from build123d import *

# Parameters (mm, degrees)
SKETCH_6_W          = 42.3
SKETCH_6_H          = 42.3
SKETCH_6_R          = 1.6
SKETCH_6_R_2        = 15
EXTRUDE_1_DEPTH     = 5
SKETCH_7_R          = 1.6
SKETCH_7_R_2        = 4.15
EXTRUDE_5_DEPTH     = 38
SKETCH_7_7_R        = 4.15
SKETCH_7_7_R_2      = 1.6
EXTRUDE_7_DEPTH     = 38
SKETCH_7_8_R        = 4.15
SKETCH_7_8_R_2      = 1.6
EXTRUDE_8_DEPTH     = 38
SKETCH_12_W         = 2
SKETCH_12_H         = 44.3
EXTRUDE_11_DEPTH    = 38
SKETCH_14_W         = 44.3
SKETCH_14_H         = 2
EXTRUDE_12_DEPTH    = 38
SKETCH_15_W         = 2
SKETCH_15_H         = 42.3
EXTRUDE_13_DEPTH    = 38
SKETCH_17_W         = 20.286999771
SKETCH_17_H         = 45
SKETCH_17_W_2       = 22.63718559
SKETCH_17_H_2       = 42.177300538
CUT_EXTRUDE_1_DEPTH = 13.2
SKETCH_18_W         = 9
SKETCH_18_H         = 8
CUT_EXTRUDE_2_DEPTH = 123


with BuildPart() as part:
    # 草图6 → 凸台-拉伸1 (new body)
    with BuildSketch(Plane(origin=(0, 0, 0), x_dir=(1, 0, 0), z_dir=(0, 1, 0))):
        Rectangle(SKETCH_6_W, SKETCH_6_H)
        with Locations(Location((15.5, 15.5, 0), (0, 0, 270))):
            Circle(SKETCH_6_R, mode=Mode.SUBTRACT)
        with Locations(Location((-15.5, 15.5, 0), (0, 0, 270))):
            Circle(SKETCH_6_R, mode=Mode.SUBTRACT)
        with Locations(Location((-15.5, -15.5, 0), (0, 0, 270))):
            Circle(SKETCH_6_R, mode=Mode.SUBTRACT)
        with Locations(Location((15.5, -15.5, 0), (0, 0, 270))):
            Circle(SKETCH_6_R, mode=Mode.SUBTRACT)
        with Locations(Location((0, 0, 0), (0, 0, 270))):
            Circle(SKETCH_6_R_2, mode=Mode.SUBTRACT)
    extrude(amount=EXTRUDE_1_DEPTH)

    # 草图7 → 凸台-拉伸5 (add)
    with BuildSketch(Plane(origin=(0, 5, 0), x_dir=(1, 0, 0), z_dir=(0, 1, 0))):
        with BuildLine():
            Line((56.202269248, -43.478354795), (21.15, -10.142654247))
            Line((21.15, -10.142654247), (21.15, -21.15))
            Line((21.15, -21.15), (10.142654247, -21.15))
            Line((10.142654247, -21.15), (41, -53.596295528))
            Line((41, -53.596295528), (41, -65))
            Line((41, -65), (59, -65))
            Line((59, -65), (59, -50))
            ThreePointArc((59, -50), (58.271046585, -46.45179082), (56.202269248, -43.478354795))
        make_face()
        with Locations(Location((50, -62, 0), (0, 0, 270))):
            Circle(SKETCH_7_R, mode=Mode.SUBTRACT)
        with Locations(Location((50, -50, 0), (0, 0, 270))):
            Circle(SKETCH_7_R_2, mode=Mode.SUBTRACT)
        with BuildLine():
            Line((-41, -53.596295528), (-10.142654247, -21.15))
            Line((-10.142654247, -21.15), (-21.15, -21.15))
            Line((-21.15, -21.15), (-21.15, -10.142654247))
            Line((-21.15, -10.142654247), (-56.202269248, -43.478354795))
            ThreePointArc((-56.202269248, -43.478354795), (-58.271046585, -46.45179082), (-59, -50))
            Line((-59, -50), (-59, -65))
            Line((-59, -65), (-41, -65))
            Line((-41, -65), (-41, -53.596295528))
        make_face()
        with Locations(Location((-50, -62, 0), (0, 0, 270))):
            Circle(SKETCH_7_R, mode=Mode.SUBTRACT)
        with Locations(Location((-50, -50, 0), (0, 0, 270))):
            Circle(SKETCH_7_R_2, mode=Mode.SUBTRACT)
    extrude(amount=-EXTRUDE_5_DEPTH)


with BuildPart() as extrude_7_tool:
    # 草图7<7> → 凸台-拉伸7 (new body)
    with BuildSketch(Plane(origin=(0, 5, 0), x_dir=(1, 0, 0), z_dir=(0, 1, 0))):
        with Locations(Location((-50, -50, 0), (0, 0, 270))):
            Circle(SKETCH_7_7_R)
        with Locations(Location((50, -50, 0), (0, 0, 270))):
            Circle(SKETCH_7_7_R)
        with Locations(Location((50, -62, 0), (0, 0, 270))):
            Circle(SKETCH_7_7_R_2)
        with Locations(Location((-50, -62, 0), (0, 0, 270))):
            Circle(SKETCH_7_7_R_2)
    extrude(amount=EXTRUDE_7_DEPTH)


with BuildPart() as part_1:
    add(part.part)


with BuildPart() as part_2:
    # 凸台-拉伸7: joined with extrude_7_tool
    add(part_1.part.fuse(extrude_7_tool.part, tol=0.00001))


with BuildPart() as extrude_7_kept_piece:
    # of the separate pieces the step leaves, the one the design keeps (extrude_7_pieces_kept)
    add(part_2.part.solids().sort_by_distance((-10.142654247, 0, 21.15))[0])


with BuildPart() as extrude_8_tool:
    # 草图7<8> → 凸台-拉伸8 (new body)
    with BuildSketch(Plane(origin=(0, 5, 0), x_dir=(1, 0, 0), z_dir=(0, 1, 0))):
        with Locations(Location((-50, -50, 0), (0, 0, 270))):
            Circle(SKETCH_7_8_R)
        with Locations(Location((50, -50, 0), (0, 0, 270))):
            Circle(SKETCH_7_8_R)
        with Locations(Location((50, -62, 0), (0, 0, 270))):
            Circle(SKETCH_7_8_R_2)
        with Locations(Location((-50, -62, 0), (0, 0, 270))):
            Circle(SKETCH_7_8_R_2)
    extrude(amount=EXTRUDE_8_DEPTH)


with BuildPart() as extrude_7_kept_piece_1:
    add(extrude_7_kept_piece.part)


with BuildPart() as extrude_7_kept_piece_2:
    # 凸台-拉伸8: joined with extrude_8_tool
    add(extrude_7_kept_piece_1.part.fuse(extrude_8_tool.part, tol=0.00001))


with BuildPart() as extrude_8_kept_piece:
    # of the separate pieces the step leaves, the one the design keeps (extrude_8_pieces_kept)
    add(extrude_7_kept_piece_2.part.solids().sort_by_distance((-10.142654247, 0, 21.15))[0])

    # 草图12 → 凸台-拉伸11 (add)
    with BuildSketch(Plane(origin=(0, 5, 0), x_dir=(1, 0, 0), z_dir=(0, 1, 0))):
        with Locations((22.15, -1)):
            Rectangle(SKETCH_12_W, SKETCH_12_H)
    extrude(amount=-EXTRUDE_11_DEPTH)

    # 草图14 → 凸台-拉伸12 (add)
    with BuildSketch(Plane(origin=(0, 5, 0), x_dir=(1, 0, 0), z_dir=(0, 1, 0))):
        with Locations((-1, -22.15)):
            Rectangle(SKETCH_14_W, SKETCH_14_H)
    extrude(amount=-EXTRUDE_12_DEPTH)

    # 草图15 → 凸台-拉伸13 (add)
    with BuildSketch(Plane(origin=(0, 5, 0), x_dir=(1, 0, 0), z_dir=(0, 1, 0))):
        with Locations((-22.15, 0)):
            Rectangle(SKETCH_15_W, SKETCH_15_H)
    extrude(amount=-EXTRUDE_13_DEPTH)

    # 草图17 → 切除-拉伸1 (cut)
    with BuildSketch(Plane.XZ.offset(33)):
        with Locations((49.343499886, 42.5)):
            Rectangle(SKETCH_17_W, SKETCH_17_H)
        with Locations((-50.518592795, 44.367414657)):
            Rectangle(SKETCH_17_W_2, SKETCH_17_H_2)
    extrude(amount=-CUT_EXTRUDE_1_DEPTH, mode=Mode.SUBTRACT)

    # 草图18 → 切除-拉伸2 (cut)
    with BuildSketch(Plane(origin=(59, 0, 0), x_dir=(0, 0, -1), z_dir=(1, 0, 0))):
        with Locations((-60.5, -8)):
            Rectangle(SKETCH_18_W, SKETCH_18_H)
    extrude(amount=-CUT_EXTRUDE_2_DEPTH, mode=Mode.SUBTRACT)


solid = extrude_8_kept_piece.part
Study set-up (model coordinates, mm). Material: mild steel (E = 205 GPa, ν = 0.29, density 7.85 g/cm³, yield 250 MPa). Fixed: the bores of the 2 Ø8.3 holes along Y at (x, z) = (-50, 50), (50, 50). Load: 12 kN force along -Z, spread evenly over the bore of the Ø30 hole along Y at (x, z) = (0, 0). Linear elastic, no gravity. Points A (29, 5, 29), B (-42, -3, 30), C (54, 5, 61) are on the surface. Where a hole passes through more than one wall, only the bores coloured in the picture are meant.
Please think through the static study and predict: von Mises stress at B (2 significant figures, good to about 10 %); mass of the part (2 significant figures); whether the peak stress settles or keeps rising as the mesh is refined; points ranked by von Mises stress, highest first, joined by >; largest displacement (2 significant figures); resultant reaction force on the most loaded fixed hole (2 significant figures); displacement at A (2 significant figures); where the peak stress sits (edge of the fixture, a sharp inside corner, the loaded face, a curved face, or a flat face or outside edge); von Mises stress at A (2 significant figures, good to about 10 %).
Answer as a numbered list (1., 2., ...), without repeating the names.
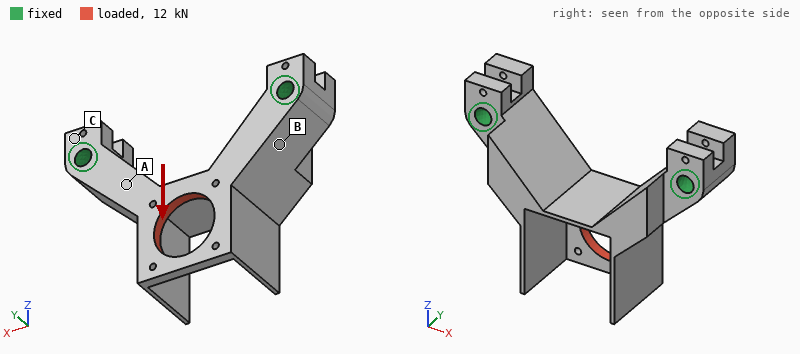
1. 27 MPa
2. 550 g
3. keeps rising
4. A > B > C
5. 63 µm
6. 8.0 kN
7. 12 µm
8. a sharp inside corner
9. 56 MPa
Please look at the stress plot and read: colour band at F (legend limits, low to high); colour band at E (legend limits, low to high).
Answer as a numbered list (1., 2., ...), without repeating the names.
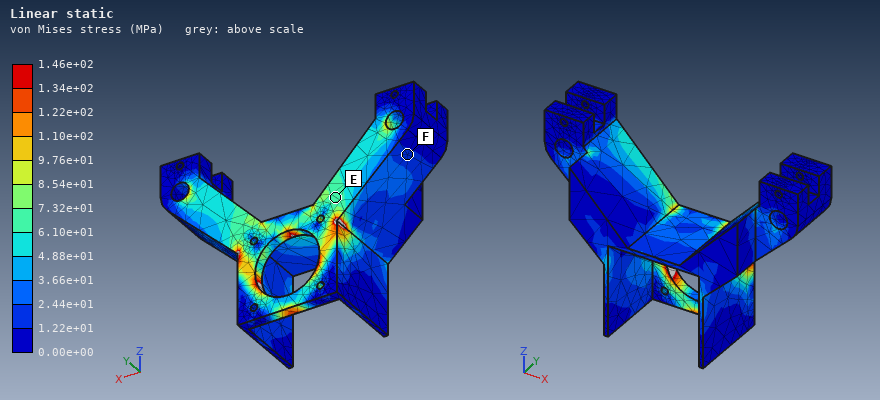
1. 1.22e+01 to 2.44e+01 MPa
2. 6.10e+01 to 7.32e+01 MPa
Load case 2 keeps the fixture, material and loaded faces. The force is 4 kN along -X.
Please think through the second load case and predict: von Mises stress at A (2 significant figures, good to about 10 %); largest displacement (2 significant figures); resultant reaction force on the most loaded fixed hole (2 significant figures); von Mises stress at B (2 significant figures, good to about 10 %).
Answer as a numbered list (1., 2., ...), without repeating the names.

1. 13 MPa
2. 43 µm
3. 2.7 kN
4. 16 MPa
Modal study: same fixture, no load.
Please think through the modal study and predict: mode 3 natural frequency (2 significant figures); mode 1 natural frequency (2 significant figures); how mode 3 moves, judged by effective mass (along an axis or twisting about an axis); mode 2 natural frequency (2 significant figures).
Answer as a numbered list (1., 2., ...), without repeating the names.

1. 4300 Hz
2. 2700 Hz
3. along Y
4. 2700 Hz
